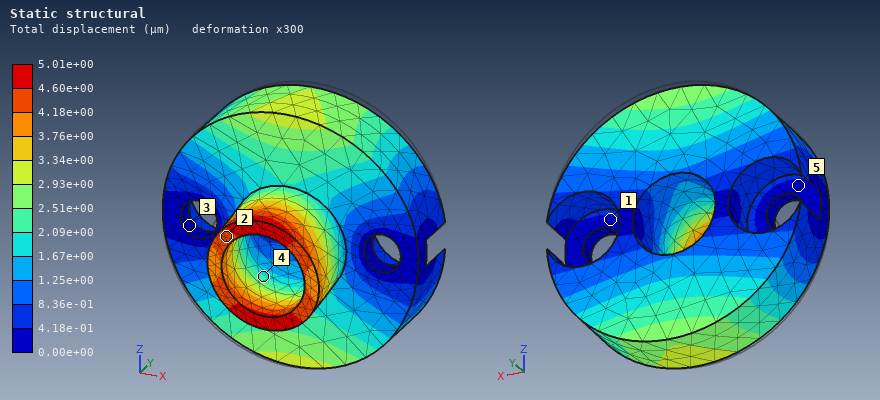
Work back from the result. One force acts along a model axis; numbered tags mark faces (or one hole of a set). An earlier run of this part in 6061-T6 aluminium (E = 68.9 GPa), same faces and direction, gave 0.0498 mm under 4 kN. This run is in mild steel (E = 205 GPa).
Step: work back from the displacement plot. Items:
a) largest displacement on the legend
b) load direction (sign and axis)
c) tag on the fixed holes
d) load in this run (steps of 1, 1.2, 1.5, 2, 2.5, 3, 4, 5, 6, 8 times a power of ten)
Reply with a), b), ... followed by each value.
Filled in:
a) 5.01e+00 µm
b) -Z
c) 3
d) 1.2 kN
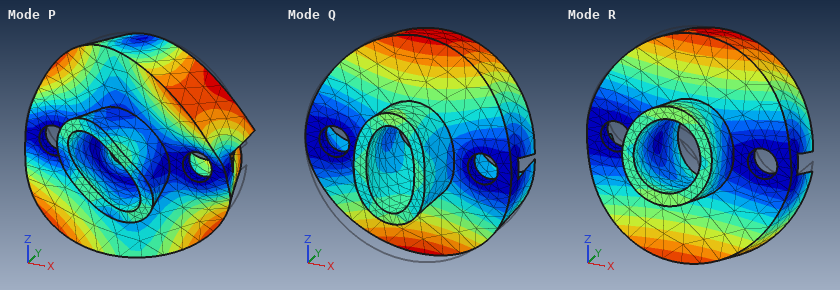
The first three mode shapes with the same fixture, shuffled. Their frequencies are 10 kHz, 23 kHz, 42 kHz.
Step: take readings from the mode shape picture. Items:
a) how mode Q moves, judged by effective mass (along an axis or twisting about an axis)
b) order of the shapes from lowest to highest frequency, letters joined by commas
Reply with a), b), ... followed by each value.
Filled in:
a) along Y
b) R, Q, P
